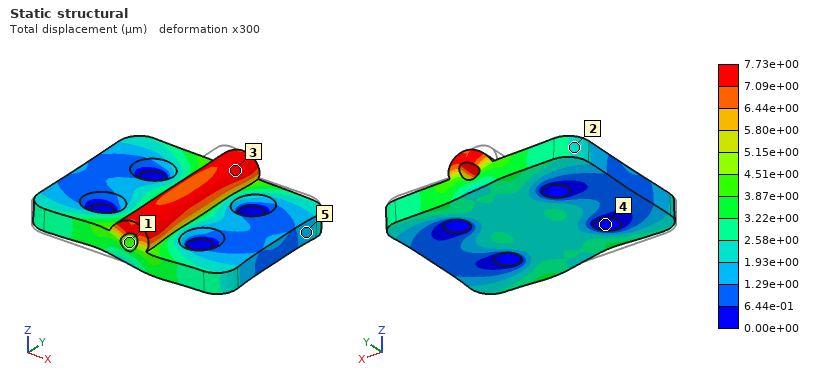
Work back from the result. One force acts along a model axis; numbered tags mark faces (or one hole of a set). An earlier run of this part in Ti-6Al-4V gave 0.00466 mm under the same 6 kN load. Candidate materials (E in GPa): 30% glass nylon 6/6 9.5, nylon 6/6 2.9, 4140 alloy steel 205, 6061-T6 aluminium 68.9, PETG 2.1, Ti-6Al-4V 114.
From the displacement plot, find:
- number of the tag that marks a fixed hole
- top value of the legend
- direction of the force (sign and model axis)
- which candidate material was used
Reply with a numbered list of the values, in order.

1. 4
2. 7.73e+00 µm
3. +X
4. 6061-T6 aluminium
